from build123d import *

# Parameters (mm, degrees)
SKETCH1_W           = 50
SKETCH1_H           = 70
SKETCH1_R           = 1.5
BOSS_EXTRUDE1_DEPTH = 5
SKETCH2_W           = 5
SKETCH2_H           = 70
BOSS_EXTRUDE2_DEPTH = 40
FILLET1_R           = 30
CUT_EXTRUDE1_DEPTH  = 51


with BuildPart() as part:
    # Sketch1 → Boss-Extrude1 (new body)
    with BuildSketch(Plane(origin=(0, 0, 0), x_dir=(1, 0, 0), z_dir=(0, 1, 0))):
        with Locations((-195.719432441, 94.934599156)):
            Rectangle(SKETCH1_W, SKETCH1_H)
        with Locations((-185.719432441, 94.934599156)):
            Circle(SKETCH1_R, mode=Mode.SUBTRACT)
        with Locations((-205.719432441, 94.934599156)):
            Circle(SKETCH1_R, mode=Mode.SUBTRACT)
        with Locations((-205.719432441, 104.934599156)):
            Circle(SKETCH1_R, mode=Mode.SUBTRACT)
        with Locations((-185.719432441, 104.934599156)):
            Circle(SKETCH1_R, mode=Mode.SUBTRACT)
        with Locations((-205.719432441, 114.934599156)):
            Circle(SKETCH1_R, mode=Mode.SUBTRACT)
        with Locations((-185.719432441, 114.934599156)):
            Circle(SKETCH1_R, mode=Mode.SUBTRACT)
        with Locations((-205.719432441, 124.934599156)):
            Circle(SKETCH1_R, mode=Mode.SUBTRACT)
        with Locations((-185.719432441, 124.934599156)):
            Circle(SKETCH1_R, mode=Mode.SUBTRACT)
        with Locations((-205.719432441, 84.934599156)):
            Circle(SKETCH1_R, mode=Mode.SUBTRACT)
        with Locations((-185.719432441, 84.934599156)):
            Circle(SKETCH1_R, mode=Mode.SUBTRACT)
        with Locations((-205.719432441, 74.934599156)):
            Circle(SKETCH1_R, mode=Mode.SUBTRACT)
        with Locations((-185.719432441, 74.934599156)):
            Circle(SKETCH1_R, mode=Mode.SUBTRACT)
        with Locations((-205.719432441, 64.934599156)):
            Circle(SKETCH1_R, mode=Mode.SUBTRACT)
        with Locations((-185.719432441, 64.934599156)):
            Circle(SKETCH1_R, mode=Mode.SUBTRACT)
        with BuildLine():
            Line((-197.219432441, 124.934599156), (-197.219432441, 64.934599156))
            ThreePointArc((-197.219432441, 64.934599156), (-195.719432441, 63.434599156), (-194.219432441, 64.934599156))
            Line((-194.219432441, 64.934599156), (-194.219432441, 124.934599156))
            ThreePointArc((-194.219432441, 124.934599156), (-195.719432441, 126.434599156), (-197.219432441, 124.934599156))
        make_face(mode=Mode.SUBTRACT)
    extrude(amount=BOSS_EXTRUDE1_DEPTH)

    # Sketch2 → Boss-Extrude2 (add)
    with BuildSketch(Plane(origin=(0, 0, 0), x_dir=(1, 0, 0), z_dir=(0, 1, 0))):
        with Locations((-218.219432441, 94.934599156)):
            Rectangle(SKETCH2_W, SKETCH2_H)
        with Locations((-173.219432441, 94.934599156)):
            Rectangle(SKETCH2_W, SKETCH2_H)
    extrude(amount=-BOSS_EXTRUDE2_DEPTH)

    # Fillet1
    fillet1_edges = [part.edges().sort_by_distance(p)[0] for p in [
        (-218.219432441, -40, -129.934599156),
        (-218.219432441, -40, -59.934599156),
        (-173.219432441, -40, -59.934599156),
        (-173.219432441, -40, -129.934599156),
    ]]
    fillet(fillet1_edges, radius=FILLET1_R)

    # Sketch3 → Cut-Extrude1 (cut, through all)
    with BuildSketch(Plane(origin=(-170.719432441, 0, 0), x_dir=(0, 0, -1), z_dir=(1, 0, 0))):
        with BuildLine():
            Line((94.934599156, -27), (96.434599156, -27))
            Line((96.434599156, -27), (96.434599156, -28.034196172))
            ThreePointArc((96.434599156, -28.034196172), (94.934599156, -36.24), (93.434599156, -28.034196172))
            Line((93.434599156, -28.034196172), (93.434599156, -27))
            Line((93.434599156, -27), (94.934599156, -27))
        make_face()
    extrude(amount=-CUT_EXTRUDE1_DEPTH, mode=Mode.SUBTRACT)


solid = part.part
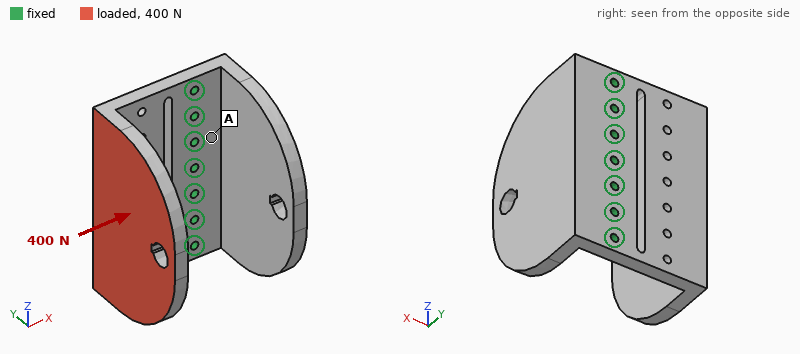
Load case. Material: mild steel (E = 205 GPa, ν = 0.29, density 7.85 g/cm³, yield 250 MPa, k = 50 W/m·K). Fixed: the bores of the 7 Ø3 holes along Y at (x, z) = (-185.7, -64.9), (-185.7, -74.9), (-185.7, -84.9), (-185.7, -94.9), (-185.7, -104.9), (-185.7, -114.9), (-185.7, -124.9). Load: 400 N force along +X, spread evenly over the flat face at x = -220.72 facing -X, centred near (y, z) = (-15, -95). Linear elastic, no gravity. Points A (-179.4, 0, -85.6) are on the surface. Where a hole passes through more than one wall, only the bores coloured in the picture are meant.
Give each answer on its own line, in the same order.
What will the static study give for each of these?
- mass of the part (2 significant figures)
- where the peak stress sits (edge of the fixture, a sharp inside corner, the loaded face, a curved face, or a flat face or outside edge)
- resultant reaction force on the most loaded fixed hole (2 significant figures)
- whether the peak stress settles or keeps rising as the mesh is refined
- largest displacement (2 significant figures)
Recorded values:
310 g
a sharp inside corner
240 N
keeps rising
0.32 mm
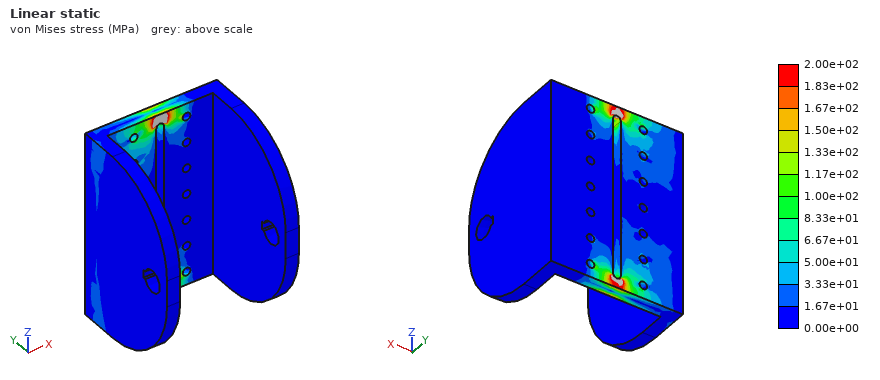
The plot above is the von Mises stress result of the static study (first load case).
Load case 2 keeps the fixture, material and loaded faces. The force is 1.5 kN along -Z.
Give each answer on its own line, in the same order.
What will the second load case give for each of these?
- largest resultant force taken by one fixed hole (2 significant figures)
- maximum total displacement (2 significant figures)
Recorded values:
1.1 kN
99 µm
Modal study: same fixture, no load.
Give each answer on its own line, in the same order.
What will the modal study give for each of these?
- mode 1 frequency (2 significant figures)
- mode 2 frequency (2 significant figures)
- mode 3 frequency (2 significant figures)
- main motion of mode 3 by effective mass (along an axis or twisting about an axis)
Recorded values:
520 Hz
1800 Hz
2000 Hz
along X
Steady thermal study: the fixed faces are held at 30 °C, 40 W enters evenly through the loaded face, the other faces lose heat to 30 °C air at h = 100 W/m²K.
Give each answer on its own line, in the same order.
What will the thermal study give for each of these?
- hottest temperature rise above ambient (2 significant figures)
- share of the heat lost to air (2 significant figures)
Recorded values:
66 K
87 %
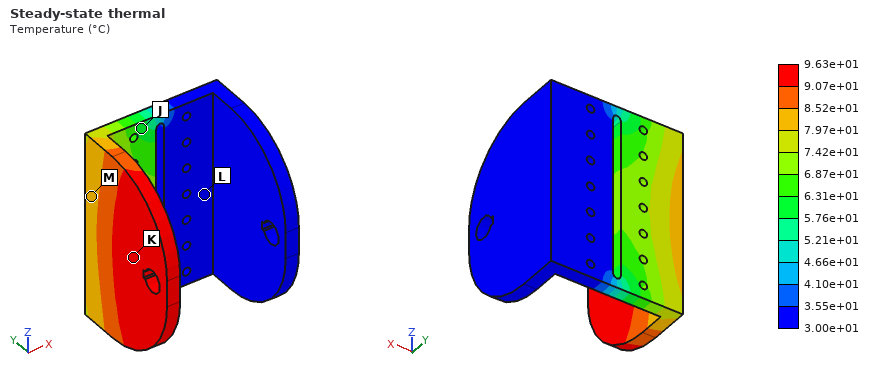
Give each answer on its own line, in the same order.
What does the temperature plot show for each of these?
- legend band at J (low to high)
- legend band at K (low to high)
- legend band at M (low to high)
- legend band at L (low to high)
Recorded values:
5.76e+01 to 6.31e+01 °C
9.07e+01 to 9.63e+01 °C
7.97e+01 to 8.52e+01 °C
3.00e+01 to 3.55e+01 °C
